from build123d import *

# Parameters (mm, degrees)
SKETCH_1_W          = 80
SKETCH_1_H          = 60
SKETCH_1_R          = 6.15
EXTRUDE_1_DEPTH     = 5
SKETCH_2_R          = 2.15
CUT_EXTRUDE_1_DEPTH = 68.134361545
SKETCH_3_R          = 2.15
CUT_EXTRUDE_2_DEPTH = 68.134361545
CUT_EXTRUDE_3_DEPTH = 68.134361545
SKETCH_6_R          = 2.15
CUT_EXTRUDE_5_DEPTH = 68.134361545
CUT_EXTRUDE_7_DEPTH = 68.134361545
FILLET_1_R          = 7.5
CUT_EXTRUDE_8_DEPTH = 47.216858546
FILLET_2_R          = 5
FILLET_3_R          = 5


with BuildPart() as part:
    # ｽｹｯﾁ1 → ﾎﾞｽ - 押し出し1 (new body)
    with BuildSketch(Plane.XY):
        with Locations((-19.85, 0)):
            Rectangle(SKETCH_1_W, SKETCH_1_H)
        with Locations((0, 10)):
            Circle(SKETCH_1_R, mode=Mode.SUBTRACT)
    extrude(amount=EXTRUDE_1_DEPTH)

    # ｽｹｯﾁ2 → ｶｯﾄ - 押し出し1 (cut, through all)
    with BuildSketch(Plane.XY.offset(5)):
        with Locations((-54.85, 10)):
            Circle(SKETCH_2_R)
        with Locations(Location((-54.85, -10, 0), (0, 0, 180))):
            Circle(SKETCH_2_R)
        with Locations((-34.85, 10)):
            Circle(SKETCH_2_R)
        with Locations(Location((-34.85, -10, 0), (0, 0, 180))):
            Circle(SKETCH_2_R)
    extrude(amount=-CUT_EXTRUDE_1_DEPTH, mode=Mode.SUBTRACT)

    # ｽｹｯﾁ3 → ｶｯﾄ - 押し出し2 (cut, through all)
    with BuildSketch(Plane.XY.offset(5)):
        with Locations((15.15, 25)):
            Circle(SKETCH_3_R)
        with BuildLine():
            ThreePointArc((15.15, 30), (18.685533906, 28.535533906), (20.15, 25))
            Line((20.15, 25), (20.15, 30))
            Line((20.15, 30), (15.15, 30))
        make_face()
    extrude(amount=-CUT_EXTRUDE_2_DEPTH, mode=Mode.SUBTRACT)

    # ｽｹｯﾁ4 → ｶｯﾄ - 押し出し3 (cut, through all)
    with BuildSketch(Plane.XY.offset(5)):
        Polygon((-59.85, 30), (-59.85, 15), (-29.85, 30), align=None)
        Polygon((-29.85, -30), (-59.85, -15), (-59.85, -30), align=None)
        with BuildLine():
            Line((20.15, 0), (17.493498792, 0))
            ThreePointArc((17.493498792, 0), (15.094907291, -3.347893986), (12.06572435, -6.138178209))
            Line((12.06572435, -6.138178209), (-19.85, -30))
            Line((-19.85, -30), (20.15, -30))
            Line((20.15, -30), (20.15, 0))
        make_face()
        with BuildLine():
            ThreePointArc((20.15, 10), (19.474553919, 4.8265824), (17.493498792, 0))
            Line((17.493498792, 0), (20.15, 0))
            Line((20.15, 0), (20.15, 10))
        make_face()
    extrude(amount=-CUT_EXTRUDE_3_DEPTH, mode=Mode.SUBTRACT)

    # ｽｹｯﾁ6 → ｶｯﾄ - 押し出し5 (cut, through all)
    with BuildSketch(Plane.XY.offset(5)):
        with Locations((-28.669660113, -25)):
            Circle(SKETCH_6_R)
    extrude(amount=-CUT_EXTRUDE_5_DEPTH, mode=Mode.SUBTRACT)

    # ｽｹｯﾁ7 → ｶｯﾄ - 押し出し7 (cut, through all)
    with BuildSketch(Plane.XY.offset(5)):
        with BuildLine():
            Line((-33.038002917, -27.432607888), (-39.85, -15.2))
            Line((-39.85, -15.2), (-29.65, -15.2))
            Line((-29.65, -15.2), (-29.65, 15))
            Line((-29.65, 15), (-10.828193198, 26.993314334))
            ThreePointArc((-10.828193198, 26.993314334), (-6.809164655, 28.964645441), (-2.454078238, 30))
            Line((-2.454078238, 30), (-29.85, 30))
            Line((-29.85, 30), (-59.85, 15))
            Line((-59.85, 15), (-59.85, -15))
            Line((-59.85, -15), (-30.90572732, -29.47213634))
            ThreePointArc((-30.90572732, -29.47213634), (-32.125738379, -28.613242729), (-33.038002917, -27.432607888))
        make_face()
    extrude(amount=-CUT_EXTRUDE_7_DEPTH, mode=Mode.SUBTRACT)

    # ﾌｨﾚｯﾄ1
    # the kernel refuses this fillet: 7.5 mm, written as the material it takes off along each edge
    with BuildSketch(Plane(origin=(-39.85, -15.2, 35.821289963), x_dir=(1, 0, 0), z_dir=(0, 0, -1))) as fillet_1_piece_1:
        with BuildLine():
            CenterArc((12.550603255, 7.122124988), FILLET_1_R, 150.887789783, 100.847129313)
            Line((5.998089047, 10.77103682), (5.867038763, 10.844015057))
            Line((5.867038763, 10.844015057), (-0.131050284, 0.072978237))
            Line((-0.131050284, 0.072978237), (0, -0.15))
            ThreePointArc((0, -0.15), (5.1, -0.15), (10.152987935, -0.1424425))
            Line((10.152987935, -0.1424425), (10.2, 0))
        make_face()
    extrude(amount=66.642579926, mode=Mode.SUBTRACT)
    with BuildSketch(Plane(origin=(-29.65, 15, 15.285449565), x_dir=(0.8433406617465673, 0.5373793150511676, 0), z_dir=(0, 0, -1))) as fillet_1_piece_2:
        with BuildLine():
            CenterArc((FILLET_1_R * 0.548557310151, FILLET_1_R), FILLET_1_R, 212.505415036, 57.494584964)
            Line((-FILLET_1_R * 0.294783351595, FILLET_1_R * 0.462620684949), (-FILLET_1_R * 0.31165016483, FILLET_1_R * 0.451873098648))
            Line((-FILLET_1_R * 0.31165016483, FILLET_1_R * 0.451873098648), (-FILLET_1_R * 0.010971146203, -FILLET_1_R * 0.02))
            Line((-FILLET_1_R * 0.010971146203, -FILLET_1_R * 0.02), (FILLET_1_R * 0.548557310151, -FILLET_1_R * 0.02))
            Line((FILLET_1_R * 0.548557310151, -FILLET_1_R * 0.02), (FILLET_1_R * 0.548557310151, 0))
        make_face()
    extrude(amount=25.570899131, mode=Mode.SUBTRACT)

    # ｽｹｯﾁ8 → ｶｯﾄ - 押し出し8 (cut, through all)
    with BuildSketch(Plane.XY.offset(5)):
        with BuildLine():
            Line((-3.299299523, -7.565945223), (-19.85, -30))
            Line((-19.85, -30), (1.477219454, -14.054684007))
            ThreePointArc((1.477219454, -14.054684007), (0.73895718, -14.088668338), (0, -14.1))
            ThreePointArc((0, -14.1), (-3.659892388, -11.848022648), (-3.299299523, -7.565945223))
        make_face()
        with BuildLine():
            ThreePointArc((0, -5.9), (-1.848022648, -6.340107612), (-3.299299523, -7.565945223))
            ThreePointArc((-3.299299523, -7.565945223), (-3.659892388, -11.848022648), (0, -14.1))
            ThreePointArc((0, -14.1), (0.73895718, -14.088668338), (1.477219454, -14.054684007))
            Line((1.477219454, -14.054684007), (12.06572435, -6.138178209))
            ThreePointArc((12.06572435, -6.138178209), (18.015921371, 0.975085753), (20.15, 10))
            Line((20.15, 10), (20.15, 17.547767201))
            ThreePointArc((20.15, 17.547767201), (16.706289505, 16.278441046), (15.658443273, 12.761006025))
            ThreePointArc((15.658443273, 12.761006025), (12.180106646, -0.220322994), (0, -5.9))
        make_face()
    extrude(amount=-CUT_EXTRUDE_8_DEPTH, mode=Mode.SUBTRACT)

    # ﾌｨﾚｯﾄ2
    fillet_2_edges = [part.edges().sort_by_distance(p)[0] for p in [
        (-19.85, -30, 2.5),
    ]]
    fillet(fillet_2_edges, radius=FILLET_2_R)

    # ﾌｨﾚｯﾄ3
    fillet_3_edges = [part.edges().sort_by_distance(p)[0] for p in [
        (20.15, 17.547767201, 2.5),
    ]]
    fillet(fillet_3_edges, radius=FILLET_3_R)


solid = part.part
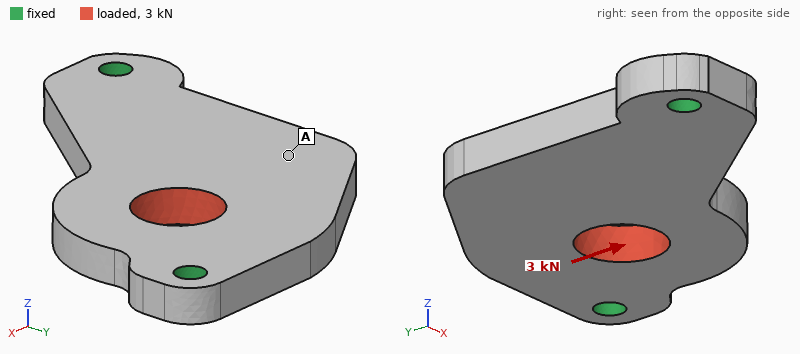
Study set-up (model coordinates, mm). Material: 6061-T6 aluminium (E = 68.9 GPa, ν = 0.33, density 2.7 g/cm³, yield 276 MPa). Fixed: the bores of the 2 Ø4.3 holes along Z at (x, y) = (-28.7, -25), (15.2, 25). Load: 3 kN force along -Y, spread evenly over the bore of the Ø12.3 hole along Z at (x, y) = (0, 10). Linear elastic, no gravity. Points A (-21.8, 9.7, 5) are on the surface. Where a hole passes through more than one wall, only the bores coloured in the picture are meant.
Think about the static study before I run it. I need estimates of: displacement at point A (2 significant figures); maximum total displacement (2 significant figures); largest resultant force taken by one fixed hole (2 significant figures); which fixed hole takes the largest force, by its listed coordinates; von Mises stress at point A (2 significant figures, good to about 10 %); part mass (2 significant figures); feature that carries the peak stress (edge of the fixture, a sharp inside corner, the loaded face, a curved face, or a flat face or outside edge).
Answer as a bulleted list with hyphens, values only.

- 14 µm
- 19 µm
- 1.6 kN
- (15.2, 25)
- 15 MPa
- 24 g
- edge of the fixture
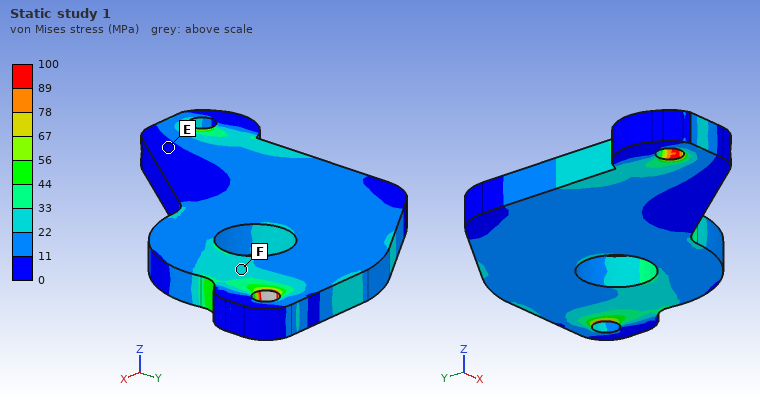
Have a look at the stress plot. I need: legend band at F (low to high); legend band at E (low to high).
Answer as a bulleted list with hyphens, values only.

- 22 to 33 MPa
- 0 to 11 MPa
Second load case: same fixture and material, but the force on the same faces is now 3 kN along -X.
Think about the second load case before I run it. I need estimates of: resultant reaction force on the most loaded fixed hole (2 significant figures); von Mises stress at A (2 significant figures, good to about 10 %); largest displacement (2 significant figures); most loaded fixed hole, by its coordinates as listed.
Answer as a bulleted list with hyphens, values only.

- 2.3 kN
- 17 MPa
- 21 µm
- (15.2, 25)
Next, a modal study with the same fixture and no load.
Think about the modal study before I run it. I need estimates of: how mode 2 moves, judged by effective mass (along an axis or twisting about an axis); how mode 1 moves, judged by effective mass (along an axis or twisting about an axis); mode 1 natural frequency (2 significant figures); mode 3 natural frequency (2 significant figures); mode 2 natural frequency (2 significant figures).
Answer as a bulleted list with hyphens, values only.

- along Z
- along Z
- 3700 Hz
- 12 kHz
- 6100 Hz
